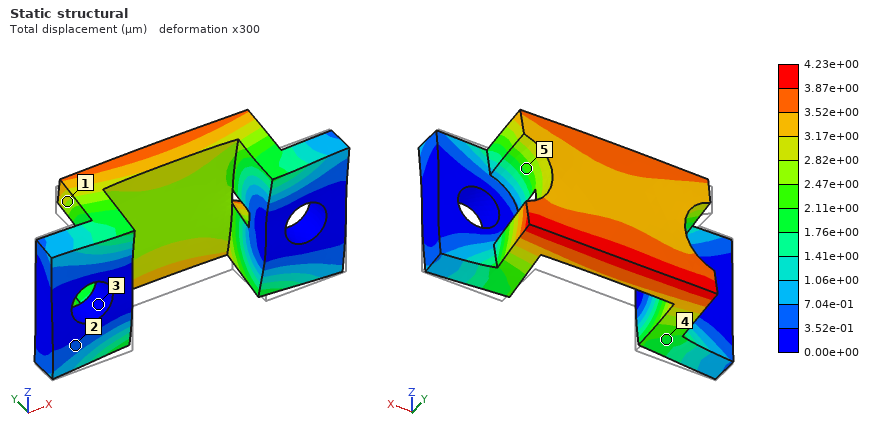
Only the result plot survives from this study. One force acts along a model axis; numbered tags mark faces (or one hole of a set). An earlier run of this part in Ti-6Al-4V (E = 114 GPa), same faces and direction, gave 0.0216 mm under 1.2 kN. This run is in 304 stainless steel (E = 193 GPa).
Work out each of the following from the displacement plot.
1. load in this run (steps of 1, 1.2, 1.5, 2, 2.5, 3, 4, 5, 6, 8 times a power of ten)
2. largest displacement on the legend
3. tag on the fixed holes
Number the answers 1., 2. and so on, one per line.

1. 400 N
2. 4.23e+00 µm
3. 3
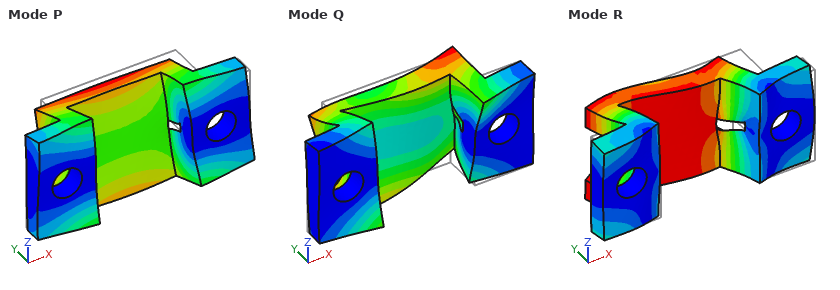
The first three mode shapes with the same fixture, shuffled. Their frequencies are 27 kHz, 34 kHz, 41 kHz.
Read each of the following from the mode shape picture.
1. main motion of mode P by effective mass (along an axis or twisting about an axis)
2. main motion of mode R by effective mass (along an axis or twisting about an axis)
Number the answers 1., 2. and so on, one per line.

1. along Z
2. along X
